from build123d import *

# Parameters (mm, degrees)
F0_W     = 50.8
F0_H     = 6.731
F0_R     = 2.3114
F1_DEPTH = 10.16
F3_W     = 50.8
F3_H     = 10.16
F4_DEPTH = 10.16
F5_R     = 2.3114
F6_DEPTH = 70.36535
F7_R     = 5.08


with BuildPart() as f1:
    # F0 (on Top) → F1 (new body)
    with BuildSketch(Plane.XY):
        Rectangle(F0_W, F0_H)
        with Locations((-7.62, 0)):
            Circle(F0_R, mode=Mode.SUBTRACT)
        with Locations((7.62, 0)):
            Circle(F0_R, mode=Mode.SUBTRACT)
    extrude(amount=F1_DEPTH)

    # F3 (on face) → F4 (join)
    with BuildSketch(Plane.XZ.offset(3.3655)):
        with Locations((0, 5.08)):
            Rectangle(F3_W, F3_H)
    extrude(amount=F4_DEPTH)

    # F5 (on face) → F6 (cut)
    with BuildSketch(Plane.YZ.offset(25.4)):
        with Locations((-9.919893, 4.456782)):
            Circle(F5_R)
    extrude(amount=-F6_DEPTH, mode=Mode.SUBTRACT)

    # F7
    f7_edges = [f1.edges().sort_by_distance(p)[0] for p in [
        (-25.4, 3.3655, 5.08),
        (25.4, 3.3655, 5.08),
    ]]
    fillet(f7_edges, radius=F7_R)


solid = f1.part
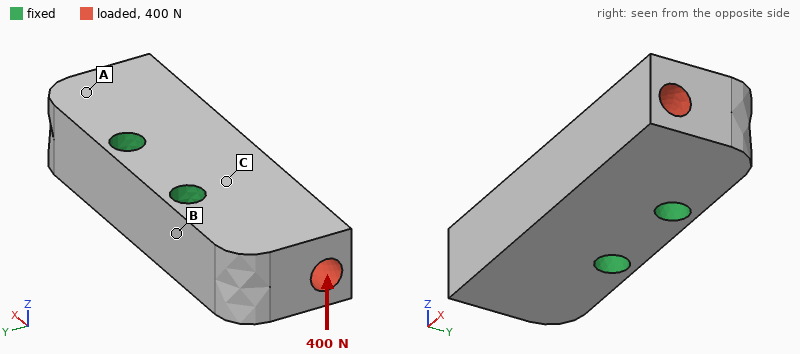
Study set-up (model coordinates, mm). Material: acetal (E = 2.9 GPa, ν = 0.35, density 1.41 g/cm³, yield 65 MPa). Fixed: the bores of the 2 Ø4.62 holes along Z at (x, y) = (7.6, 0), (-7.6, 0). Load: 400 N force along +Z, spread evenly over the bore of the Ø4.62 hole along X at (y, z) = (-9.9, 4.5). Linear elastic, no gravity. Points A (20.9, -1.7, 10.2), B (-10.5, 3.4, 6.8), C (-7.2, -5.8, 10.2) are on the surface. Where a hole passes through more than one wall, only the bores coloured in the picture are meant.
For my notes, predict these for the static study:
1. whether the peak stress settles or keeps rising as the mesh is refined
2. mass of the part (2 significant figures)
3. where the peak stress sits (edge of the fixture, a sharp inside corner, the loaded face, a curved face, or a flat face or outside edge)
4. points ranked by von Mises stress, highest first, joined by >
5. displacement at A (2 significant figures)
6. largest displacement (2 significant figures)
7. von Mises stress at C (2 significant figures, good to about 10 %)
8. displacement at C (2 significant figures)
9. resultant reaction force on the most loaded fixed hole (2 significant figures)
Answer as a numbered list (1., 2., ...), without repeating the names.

1. keeps rising
2. 10 g
3. edge of the fixture
4. C > B > A
5. 29 µm
6. 83 µm
7. 4.6 MPa
8. 16 µm
9. 200 N
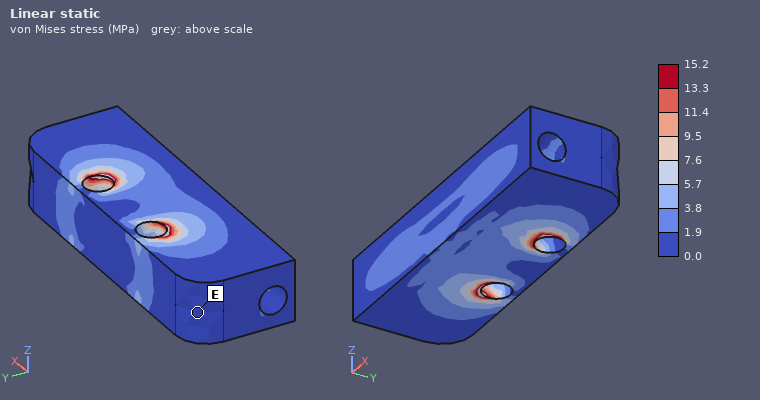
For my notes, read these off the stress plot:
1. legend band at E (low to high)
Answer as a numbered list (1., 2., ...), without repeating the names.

1. 0.0 to 1.9 MPa
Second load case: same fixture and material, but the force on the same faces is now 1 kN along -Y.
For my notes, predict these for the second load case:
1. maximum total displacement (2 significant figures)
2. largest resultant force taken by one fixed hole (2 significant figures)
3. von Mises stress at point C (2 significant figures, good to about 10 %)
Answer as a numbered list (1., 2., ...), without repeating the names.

1. 76 µm
2. 520 N
3. 3.3 MPa
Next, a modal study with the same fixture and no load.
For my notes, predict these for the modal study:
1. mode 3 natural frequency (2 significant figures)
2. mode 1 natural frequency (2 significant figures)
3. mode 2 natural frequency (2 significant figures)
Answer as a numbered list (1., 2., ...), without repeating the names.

1. 5800 Hz
2. 5600 Hz
3. 5800 Hz
